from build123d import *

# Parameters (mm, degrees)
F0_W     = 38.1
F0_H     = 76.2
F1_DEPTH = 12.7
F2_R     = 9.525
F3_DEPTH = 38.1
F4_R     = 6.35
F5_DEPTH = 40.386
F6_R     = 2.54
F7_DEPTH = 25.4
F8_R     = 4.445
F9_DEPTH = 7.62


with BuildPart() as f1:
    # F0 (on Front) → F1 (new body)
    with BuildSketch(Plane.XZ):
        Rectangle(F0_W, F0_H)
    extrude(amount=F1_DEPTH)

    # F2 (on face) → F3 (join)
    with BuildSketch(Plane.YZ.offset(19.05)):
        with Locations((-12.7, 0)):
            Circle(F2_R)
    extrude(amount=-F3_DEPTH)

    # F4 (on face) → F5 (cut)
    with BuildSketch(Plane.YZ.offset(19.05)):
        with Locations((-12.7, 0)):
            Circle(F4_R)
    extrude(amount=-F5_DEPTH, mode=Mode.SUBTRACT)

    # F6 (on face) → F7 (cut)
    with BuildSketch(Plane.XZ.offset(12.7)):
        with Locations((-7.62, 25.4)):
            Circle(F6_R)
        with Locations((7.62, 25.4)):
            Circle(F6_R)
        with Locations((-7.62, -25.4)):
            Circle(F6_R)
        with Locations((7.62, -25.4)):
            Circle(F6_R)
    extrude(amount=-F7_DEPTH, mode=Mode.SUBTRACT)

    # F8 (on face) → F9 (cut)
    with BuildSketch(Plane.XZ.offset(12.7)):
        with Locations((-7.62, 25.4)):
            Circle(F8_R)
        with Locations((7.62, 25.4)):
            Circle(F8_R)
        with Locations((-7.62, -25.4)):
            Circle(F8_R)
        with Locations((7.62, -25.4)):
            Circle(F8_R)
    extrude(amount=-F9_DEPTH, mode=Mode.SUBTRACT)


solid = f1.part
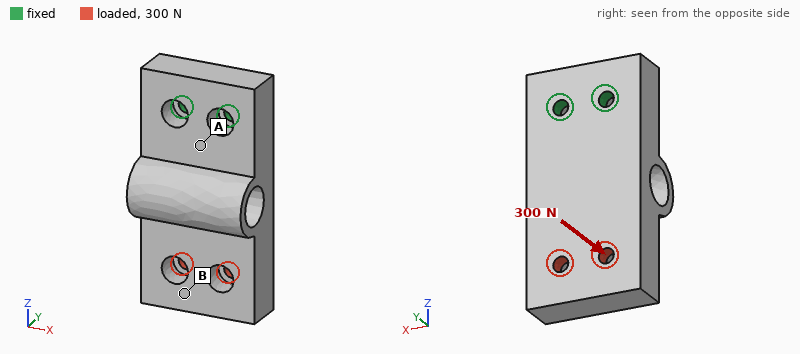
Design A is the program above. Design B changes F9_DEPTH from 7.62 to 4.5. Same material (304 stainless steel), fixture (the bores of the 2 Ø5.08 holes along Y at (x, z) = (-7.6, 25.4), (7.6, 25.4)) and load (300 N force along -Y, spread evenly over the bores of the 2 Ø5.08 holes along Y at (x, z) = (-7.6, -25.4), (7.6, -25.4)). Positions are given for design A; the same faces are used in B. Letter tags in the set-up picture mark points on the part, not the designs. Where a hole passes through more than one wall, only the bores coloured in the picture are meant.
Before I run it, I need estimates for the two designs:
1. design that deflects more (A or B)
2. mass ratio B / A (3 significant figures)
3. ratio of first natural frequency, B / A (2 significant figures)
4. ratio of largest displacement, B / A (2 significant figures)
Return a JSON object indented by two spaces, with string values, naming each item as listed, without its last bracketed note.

{
  "design that deflects more": "A",
  "mass ratio B / A": "1.01",
  "ratio of first natural frequency, B / A": "1.2",
  "ratio of largest displacement, B / A": "0.67"
}
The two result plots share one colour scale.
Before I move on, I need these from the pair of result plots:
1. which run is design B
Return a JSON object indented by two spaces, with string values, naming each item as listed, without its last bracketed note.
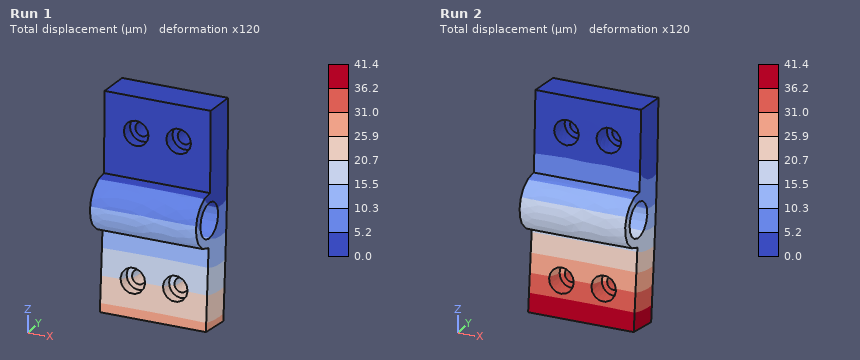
{
  "which run is design B": "Run 1"
}
